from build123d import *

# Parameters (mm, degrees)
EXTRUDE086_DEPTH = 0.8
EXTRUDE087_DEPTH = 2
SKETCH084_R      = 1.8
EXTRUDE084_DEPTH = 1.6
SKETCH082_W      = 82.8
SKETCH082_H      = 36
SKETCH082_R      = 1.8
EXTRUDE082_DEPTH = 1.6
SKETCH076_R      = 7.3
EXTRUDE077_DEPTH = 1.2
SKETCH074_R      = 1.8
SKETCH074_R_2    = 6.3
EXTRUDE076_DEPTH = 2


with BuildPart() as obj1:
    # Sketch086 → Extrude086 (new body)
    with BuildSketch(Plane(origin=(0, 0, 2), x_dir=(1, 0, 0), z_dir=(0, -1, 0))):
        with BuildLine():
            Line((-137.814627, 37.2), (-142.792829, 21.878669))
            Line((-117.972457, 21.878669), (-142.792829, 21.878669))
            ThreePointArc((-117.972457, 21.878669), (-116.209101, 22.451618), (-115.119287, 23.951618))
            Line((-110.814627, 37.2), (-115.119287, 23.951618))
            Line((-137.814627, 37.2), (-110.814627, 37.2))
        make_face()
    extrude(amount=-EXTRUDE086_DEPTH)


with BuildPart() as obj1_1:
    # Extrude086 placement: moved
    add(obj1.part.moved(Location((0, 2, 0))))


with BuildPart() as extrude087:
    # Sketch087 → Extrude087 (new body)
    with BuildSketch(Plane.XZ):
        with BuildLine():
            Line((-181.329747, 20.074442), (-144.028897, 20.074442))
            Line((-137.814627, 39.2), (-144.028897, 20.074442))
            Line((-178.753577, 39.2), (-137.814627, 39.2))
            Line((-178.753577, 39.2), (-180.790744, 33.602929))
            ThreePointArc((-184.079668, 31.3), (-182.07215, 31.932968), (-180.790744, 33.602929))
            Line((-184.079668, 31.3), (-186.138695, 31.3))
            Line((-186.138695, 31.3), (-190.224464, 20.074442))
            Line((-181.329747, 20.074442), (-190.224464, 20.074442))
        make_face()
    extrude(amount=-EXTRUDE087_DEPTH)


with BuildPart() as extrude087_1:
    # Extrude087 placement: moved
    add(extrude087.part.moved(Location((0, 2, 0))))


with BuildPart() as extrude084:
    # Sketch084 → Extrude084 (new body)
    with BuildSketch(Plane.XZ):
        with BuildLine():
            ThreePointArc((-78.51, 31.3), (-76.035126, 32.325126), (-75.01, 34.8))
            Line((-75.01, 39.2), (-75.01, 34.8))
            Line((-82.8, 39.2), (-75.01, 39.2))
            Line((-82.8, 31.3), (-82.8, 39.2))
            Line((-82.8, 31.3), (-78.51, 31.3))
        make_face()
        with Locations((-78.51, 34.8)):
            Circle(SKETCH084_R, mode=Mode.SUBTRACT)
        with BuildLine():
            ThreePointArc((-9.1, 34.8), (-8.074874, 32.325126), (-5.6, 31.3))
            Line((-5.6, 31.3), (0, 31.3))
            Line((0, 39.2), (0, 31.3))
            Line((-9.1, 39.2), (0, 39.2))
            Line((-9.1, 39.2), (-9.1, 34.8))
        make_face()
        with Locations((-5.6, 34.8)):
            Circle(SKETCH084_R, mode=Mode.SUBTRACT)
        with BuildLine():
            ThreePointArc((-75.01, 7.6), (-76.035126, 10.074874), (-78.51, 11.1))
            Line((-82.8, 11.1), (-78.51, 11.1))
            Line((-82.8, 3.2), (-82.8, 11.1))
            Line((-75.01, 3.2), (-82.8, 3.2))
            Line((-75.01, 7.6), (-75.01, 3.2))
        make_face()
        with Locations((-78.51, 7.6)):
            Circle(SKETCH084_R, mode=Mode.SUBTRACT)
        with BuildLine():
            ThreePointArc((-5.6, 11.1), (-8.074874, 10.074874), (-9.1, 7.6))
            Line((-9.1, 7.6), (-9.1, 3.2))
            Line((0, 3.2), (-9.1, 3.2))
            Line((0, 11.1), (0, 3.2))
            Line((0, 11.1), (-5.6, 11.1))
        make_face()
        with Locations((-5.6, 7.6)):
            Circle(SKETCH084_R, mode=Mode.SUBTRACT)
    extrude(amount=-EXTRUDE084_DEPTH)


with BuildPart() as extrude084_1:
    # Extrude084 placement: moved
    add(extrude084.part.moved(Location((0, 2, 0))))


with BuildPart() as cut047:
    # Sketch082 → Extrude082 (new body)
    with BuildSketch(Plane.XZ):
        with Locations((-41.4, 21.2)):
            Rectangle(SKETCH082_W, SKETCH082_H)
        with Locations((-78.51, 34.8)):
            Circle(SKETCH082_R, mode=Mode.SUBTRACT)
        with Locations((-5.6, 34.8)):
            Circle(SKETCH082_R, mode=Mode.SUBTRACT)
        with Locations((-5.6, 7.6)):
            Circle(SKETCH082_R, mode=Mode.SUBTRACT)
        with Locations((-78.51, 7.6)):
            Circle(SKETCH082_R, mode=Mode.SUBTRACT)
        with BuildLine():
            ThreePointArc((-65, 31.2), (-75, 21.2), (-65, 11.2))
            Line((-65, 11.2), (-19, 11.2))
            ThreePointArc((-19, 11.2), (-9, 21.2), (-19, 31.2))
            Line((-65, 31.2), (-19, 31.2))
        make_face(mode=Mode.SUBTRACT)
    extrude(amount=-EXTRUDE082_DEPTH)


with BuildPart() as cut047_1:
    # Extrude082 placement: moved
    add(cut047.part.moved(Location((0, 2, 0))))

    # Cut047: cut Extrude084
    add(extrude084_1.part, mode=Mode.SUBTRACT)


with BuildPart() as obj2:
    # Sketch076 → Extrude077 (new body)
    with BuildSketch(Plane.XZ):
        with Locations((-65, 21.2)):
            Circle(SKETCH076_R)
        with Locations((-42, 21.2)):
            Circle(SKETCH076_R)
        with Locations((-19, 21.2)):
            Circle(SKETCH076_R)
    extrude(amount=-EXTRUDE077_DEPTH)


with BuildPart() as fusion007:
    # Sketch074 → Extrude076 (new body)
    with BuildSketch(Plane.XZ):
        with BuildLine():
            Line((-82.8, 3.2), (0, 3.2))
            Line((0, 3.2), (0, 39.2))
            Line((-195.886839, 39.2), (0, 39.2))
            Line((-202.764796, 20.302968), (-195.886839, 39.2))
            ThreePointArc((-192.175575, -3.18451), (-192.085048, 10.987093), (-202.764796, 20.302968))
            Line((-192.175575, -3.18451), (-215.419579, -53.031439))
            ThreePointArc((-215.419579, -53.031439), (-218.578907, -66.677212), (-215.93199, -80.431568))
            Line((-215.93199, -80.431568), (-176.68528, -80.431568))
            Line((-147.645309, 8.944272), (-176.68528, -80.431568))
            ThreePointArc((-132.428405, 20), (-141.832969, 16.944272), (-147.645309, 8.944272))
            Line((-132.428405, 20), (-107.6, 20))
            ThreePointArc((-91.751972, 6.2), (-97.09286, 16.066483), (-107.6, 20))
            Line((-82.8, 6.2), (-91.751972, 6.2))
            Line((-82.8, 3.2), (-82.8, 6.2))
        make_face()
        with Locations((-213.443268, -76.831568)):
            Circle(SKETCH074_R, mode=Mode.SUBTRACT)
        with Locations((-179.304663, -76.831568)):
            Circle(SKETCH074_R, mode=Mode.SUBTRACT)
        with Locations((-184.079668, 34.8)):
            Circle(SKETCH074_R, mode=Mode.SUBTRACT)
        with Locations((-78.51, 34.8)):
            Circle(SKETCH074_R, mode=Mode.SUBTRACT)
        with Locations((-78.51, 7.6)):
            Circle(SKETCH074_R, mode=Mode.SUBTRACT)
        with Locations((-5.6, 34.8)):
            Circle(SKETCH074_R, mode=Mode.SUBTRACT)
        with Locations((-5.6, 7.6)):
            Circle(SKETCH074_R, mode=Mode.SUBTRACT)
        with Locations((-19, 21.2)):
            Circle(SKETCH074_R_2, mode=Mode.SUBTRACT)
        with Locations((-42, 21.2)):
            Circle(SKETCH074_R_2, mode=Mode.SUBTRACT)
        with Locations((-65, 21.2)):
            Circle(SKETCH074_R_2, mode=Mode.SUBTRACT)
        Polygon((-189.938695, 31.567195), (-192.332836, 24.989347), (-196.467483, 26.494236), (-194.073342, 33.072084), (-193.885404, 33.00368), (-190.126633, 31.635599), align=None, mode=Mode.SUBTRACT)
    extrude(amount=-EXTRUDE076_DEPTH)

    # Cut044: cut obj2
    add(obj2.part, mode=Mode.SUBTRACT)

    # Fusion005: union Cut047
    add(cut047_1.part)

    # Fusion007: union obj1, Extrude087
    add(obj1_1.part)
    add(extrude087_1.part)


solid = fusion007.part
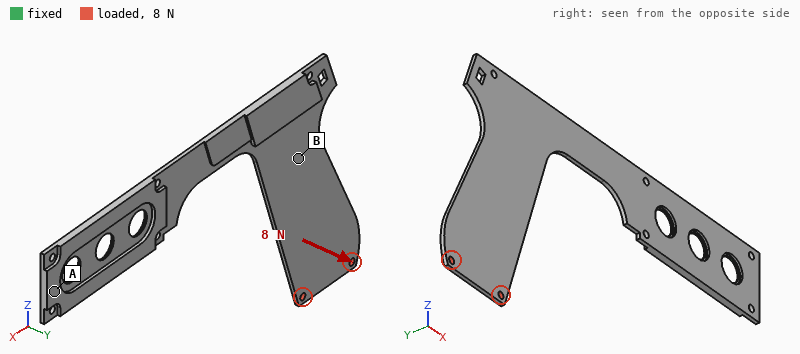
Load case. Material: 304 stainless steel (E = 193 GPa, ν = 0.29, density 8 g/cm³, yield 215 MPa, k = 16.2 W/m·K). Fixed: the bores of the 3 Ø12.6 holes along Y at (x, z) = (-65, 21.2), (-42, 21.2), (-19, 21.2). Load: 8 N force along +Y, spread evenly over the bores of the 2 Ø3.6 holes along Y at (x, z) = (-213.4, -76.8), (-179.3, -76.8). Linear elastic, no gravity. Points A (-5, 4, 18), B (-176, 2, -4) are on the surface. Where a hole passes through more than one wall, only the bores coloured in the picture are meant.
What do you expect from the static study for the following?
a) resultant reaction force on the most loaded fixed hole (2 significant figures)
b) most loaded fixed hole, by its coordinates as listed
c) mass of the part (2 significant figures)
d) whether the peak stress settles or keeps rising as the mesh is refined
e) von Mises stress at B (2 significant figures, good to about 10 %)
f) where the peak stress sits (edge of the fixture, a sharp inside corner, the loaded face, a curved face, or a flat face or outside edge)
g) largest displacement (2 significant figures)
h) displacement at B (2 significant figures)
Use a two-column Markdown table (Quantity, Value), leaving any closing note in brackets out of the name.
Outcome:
| Quantity | Value |
|---|---|
| resultant reaction force on the most loaded fixed hole | 28 N |
| most loaded fixed hole, by its coordinates as listed | (-65, 21.2) |
| mass of the part | 180 g |
| whether the peak stress settles or keeps rising as the mesh is refined | keeps rising |
| von Mises stress at B | 23 MPa |
| where the peak stress sits | edge of the fixture |
| largest displacement | 2.9 mm |
| displacement at B | 1.2 mm |
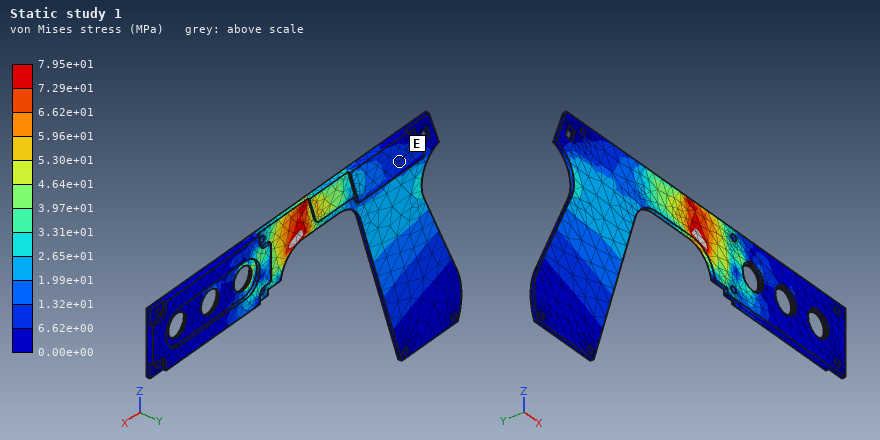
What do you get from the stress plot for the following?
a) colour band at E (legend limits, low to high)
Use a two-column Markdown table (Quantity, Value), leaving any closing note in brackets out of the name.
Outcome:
| Quantity | Value |
|---|---|
| colour band at E | 6.62e+00 to 1.32e+01 MPa |
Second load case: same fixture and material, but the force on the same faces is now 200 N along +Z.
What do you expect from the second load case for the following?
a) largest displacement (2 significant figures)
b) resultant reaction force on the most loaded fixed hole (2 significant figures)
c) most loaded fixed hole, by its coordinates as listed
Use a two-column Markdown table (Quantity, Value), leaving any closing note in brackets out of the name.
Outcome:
| Quantity | Value |
|---|---|
| largest displacement | 0.67 mm |
| resultant reaction force on the most loaded fixed hole | 650 N |
| most loaded fixed hole, by its coordinates as listed | (-65, 21.2) |
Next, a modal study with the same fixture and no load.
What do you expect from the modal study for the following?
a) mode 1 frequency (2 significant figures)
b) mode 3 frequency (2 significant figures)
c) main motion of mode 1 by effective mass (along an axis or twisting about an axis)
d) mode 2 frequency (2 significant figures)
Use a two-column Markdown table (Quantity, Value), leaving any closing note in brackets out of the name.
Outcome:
| Quantity | Value |
|---|---|
| mode 1 frequency | 44 Hz |
| mode 3 frequency | 360 Hz |
| main motion of mode 1 by effective mass | along Y |
| mode 2 frequency | 130 Hz |
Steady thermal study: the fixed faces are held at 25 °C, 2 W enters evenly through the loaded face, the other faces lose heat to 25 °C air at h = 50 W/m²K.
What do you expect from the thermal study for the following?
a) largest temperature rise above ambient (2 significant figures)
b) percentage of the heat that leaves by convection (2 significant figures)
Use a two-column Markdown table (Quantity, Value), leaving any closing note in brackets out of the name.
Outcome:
| Quantity | Value |
|---|---|
| largest temperature rise above ambient | 34 K |
| percentage of the heat that leaves by convection | 100 % |
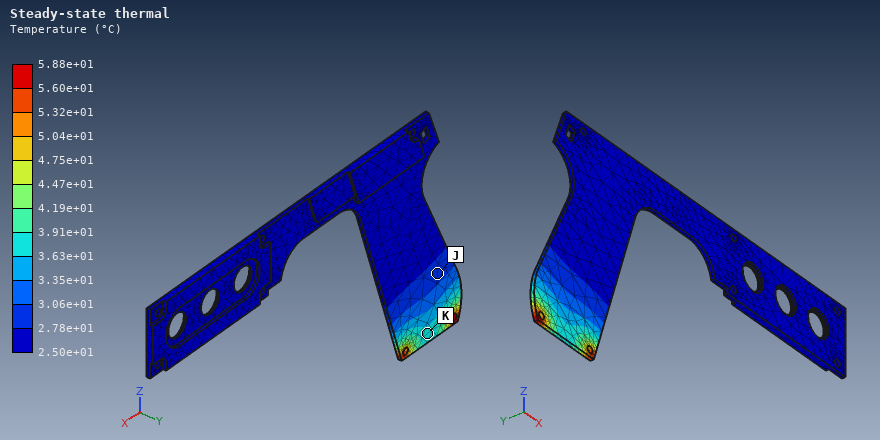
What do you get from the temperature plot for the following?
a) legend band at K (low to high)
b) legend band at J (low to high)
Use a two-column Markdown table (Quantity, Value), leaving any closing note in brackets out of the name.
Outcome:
| Quantity | Value |
|---|---|
| legend band at K | 3.63e+01 to 3.91e+01 °C |
| legend band at J | 2.78e+01 to 3.06e+01 °C |
